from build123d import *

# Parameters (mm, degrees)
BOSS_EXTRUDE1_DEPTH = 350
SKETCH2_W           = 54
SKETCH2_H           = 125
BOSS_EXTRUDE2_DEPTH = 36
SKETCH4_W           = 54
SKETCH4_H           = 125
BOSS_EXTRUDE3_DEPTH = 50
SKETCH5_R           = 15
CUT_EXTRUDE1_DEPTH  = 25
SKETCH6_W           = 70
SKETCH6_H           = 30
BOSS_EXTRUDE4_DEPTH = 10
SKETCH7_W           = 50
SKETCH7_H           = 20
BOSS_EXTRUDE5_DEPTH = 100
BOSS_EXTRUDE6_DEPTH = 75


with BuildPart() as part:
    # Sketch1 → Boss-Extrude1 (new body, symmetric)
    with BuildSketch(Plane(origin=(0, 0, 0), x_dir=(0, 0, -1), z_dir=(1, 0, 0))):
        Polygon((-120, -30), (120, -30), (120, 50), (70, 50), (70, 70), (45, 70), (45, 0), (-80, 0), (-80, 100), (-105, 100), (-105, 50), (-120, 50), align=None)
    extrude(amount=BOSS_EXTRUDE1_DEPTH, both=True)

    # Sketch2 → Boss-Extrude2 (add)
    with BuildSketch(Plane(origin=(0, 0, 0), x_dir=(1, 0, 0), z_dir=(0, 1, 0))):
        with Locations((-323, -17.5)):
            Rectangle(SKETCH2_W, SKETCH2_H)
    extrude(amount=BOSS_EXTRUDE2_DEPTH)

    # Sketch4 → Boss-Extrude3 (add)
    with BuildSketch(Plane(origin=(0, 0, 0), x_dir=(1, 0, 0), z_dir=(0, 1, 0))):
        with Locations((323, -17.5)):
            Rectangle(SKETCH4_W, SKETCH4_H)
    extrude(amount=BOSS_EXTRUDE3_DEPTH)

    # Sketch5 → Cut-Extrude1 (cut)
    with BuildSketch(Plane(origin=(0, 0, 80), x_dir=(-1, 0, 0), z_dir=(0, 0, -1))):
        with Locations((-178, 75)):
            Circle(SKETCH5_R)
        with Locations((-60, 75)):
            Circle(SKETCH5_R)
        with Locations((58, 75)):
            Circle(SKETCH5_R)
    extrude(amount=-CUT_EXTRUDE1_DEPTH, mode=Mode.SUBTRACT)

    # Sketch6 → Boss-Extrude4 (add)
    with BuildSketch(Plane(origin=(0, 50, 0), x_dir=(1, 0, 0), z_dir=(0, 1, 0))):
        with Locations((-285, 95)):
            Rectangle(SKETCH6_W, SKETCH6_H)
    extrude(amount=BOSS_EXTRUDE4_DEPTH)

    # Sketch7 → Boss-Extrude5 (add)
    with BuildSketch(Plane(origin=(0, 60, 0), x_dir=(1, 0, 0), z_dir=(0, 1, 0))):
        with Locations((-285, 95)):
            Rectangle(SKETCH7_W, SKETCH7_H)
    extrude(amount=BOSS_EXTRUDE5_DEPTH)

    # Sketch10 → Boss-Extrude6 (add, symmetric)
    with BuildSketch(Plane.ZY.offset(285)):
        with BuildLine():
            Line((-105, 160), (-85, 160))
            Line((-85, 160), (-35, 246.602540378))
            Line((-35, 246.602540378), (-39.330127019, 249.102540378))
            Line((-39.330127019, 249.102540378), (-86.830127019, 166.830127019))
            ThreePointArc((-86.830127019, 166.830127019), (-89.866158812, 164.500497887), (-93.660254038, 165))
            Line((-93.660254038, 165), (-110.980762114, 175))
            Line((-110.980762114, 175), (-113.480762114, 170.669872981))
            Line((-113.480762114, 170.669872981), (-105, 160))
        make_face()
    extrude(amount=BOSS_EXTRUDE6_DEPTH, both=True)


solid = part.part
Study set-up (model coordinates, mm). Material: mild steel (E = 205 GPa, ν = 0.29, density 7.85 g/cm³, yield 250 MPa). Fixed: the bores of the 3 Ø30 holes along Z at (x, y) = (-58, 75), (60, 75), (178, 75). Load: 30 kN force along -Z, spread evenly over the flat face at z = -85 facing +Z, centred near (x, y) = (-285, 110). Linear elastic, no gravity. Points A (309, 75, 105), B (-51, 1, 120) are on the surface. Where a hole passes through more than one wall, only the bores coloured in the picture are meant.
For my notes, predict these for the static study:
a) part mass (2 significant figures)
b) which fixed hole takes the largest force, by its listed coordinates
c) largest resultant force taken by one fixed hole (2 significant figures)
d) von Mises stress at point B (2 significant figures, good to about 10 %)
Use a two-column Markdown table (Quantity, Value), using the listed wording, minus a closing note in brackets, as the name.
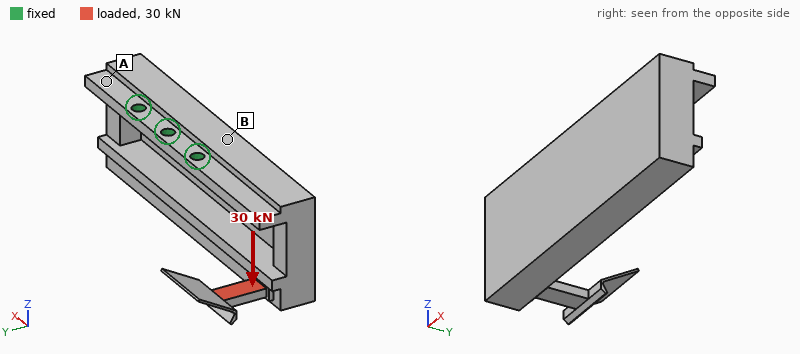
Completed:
| Quantity | Value |
|---|---|
| part mass | 87 kg |
| which fixed hole takes the largest force, by its listed coordinates | (-58, 75) |
| largest resultant force taken by one fixed hole | 54 kN |
| von Mises stress at point B | 41 MPa |
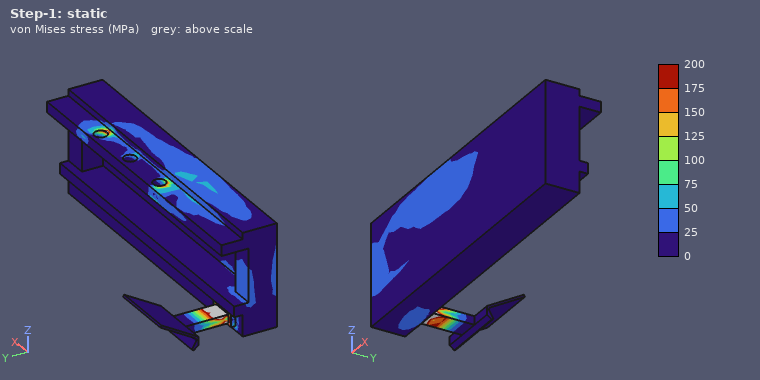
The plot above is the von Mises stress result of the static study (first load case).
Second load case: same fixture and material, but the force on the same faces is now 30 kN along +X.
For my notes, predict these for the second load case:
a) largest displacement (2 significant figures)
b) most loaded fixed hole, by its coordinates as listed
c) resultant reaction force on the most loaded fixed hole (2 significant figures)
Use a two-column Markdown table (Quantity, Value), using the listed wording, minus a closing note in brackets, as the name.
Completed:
| Quantity | Value |
|---|---|
| largest displacement | 0.72 mm |
| most loaded fixed hole, by its coordinates as listed | (-58, 75) |
| resultant reaction force on the most loaded fixed hole | 31 kN |
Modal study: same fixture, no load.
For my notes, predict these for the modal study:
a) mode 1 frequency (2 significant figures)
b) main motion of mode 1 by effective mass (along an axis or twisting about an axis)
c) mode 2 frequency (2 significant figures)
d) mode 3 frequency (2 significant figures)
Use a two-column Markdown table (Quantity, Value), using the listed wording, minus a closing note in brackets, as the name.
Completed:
| Quantity | Value |
|---|---|
| mode 1 frequency | 180 Hz |
| main motion of mode 1 by effective mass | along Y |
| mode 2 frequency | 270 Hz |
| mode 3 frequency | 310 Hz |
